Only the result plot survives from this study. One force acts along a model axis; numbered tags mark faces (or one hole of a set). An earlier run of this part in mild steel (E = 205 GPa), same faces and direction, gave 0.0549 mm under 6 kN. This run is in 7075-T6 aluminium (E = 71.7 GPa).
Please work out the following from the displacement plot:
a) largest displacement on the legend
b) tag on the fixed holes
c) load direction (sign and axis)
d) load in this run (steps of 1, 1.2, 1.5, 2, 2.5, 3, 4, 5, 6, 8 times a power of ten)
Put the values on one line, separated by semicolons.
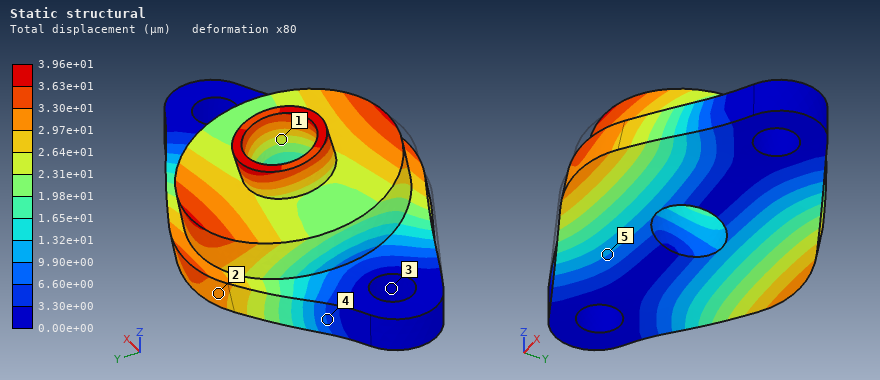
3.96e+01 µm; 3; +Y; 1.5 kN
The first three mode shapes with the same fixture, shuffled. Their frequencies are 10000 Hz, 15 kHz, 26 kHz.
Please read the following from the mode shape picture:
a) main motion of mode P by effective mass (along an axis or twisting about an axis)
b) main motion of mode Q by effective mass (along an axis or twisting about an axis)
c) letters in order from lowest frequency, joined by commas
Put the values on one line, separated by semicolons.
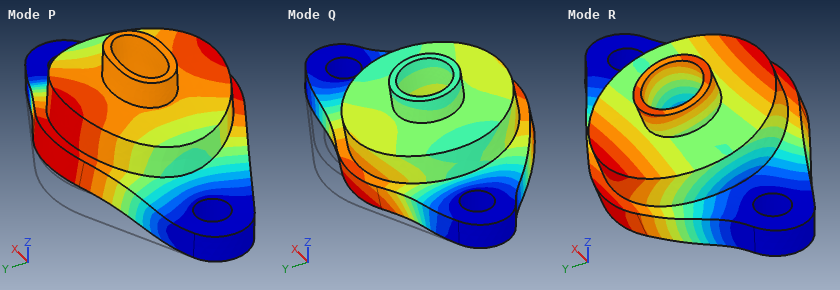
along Z; along Y; R, P, Q
